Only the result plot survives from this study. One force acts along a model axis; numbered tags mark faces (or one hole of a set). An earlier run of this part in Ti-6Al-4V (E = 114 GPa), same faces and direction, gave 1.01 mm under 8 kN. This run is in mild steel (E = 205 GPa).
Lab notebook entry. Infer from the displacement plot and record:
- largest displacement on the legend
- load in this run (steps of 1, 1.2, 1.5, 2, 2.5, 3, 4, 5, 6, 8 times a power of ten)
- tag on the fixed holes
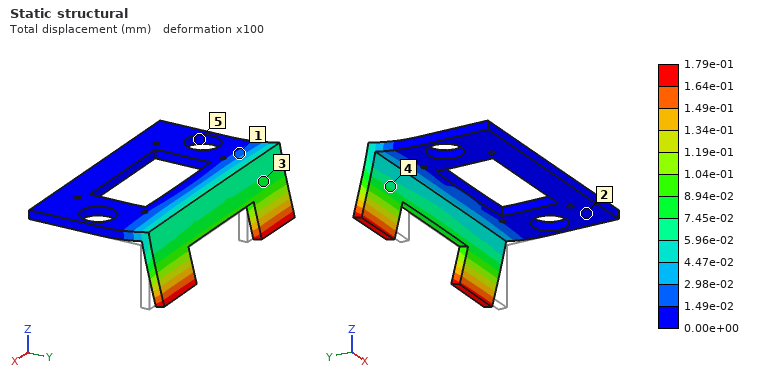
1.79e-01 mm
2.5 kN
5
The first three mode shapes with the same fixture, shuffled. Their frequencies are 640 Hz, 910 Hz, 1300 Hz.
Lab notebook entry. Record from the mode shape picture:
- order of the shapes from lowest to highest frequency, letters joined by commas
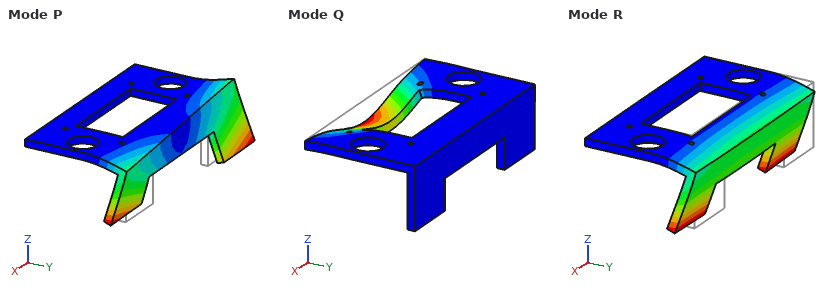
R, P, Q
